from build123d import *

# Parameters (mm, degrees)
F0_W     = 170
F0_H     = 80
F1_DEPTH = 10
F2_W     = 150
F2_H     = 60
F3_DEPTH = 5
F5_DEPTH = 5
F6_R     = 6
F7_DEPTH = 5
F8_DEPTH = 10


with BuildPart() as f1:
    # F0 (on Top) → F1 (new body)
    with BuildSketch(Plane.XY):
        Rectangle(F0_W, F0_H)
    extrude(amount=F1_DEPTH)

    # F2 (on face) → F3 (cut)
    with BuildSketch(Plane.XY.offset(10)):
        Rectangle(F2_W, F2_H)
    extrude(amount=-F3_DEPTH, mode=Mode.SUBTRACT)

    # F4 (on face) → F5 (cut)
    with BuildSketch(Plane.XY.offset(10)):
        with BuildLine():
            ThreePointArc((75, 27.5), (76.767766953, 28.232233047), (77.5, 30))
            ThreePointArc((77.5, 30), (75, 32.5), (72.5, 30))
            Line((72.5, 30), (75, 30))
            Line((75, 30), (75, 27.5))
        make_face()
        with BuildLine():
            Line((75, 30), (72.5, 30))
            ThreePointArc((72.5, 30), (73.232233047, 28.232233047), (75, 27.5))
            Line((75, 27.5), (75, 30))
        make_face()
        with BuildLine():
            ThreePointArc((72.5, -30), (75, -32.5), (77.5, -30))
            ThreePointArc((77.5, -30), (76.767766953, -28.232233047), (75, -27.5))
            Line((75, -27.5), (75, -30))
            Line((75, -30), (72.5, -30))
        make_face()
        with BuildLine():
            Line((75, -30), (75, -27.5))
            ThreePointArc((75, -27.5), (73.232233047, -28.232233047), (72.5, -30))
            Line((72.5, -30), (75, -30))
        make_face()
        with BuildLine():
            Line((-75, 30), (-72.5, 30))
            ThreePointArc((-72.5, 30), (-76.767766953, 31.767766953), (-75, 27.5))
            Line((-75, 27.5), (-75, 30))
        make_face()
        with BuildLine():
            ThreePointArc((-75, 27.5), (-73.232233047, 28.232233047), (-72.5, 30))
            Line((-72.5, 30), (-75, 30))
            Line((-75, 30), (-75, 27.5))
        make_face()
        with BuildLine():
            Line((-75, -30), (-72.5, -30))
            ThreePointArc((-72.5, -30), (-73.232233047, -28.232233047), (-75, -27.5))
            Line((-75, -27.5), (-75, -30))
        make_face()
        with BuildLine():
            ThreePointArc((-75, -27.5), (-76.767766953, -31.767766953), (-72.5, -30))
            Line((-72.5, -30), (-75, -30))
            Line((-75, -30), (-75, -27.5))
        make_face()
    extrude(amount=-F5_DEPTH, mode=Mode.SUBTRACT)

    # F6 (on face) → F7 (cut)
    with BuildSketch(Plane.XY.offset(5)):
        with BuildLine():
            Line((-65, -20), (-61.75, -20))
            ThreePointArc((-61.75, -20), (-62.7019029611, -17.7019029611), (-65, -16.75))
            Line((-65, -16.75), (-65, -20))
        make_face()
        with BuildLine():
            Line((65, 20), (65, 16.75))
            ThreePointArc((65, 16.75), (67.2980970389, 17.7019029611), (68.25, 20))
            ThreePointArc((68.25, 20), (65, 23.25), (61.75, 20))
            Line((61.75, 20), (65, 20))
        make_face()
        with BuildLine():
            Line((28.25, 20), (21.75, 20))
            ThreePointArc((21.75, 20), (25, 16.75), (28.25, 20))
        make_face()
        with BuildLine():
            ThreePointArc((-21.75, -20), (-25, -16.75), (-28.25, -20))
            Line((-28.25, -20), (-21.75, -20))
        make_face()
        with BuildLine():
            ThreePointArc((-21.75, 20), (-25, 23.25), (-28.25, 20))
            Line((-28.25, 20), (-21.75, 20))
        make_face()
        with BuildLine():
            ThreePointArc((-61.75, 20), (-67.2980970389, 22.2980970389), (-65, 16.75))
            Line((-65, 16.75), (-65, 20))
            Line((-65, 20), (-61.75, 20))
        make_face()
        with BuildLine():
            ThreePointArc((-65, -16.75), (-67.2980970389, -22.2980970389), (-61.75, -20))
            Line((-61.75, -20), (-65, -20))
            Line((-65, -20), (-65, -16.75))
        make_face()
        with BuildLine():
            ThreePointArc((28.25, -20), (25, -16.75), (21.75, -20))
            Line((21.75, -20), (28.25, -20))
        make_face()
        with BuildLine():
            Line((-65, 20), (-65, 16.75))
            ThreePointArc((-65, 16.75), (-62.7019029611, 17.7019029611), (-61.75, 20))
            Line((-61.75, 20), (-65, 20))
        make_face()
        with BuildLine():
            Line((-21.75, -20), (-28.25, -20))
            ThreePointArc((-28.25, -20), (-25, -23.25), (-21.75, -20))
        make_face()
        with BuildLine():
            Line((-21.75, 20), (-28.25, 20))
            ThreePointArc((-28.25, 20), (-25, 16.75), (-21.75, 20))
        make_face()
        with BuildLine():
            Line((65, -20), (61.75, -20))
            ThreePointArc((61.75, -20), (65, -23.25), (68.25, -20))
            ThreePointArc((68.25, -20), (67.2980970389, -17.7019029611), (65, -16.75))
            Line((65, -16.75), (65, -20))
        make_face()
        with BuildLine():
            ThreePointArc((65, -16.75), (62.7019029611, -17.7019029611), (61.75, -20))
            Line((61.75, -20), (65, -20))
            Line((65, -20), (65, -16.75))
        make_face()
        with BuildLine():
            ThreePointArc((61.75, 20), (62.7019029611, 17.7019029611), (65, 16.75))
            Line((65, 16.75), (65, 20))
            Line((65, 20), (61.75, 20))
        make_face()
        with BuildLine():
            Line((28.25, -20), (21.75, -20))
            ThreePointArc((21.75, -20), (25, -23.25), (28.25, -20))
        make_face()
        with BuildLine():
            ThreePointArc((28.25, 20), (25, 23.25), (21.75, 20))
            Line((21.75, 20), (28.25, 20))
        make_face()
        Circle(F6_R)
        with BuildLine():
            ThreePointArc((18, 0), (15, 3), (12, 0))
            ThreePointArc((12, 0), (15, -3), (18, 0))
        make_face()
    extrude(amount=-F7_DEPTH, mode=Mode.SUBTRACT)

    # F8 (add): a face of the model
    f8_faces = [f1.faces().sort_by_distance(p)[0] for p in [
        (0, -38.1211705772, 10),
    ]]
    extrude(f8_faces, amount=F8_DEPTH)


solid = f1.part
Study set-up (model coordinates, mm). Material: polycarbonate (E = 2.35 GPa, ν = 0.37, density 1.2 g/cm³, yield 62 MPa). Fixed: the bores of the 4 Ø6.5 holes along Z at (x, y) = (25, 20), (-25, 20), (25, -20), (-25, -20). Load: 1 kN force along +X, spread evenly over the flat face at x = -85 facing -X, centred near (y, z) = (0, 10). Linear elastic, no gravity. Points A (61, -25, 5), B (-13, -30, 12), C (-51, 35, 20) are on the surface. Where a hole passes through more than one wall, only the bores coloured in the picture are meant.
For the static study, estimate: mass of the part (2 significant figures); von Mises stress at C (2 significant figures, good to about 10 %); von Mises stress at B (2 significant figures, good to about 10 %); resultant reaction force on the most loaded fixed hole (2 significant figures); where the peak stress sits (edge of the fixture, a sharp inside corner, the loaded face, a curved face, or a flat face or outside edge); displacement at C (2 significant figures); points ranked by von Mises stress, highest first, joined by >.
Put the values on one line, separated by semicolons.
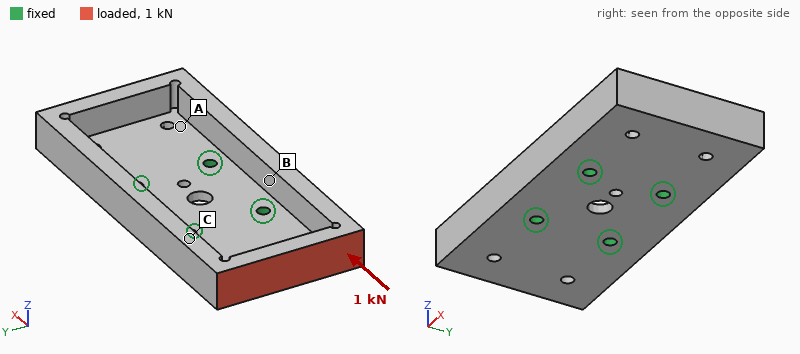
160 g; 3.8 MPa; 1.8 MPa; 340 N; a curved face; 0.16 mm; C > B > A
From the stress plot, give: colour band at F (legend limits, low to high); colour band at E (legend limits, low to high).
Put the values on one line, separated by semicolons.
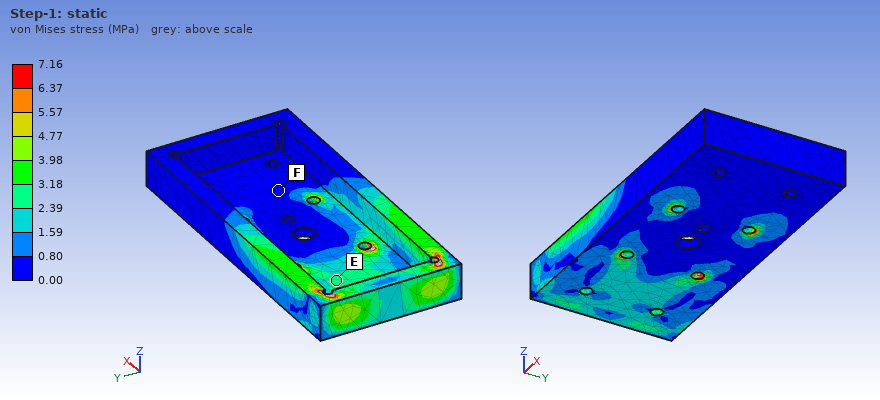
0.00 to 0.80 MPa; 2.39 to 3.18 MPa
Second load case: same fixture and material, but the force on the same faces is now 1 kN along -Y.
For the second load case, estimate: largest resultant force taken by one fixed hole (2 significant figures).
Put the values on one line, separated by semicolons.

1.1 kN
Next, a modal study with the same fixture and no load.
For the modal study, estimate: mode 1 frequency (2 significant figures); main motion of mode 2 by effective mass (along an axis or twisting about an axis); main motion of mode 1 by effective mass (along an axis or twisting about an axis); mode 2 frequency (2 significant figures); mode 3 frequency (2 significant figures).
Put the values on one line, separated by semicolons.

480 Hz; along Z; twisting about Y; 580 Hz; 630 Hz
